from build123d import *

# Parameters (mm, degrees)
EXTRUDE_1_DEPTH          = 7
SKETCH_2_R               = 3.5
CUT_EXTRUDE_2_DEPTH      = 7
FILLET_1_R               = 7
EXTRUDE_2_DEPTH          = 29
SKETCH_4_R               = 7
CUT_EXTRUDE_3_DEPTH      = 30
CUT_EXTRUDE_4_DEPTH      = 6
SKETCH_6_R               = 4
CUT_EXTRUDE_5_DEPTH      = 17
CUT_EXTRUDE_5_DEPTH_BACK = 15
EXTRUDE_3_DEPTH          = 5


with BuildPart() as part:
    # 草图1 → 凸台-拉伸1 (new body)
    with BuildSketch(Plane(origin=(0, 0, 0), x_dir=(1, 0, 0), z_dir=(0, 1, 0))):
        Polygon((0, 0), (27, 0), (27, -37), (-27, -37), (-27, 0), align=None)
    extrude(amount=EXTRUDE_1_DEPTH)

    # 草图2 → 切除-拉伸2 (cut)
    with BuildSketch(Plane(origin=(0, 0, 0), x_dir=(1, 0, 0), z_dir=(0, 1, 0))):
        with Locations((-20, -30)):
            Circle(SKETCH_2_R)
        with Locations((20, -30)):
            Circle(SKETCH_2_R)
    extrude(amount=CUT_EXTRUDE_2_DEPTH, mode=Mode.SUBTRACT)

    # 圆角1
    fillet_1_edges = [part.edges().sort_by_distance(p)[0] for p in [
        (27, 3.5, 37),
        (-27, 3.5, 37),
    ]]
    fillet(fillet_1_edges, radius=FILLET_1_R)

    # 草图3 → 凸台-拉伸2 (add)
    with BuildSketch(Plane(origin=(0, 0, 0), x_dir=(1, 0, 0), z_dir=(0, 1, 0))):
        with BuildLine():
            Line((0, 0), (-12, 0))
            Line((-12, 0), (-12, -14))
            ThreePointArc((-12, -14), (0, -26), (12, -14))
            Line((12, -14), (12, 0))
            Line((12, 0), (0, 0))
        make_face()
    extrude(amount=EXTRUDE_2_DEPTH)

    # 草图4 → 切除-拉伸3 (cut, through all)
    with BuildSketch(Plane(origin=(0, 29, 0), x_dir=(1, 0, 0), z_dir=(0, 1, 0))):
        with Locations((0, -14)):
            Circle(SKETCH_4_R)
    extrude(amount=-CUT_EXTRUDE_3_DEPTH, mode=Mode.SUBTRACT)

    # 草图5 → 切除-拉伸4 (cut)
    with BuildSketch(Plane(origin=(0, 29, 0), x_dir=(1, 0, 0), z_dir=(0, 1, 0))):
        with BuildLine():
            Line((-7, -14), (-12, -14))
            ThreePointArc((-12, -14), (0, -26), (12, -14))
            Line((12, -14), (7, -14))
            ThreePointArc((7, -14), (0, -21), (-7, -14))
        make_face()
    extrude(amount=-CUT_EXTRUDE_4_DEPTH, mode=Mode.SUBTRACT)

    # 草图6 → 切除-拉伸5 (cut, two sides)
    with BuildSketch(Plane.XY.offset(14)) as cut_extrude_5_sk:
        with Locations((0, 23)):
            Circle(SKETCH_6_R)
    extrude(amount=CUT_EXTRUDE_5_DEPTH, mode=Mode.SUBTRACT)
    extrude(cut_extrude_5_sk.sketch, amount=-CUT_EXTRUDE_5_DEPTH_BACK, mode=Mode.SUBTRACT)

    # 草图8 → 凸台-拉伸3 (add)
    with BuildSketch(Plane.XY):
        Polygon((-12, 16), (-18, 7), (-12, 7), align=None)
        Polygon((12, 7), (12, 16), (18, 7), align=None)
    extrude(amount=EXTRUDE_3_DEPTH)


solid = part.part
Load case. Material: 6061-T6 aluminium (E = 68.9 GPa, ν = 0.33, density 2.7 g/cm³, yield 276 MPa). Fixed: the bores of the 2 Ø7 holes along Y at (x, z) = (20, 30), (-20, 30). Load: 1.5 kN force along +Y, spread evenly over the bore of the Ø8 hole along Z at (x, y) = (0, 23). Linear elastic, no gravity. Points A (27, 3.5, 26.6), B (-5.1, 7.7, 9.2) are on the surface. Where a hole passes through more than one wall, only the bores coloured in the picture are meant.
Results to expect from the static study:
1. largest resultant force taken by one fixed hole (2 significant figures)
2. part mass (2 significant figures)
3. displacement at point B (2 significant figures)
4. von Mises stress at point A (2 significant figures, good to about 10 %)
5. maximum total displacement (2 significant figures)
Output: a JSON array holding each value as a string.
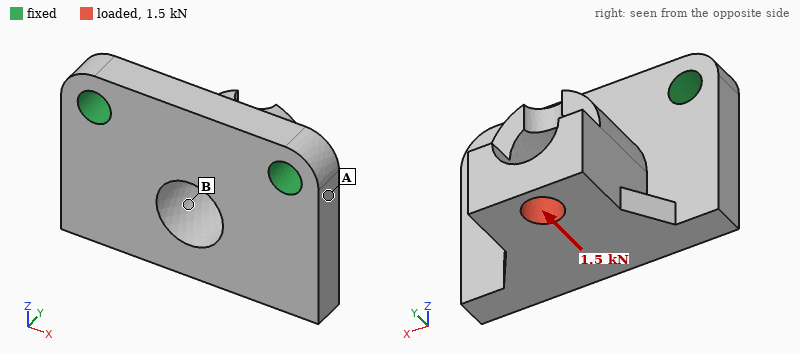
["750 N", "54 g", "0.069 mm", "35 MPa", "0.15 mm"]
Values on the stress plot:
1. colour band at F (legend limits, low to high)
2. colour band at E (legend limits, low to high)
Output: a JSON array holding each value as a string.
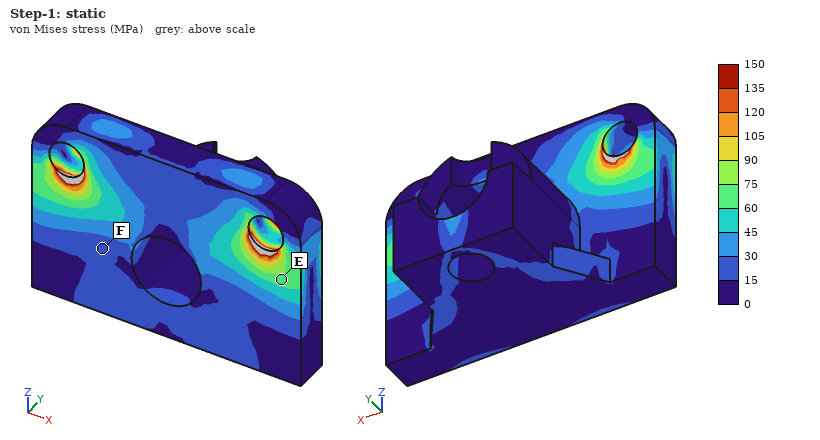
["15 to 30 MPa", "60 to 75 MPa"]
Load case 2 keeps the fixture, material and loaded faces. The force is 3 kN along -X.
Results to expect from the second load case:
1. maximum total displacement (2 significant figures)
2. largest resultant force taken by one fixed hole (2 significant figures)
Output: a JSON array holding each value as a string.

["89 µm", "2.9 kN"]
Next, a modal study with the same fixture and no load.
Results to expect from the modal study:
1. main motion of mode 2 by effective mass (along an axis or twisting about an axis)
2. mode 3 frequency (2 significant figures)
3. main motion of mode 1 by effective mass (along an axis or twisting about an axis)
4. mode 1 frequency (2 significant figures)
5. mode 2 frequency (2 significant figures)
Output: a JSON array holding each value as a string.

["along X", "14 kHz", "along Y", "3600 Hz", "8400 Hz"]
